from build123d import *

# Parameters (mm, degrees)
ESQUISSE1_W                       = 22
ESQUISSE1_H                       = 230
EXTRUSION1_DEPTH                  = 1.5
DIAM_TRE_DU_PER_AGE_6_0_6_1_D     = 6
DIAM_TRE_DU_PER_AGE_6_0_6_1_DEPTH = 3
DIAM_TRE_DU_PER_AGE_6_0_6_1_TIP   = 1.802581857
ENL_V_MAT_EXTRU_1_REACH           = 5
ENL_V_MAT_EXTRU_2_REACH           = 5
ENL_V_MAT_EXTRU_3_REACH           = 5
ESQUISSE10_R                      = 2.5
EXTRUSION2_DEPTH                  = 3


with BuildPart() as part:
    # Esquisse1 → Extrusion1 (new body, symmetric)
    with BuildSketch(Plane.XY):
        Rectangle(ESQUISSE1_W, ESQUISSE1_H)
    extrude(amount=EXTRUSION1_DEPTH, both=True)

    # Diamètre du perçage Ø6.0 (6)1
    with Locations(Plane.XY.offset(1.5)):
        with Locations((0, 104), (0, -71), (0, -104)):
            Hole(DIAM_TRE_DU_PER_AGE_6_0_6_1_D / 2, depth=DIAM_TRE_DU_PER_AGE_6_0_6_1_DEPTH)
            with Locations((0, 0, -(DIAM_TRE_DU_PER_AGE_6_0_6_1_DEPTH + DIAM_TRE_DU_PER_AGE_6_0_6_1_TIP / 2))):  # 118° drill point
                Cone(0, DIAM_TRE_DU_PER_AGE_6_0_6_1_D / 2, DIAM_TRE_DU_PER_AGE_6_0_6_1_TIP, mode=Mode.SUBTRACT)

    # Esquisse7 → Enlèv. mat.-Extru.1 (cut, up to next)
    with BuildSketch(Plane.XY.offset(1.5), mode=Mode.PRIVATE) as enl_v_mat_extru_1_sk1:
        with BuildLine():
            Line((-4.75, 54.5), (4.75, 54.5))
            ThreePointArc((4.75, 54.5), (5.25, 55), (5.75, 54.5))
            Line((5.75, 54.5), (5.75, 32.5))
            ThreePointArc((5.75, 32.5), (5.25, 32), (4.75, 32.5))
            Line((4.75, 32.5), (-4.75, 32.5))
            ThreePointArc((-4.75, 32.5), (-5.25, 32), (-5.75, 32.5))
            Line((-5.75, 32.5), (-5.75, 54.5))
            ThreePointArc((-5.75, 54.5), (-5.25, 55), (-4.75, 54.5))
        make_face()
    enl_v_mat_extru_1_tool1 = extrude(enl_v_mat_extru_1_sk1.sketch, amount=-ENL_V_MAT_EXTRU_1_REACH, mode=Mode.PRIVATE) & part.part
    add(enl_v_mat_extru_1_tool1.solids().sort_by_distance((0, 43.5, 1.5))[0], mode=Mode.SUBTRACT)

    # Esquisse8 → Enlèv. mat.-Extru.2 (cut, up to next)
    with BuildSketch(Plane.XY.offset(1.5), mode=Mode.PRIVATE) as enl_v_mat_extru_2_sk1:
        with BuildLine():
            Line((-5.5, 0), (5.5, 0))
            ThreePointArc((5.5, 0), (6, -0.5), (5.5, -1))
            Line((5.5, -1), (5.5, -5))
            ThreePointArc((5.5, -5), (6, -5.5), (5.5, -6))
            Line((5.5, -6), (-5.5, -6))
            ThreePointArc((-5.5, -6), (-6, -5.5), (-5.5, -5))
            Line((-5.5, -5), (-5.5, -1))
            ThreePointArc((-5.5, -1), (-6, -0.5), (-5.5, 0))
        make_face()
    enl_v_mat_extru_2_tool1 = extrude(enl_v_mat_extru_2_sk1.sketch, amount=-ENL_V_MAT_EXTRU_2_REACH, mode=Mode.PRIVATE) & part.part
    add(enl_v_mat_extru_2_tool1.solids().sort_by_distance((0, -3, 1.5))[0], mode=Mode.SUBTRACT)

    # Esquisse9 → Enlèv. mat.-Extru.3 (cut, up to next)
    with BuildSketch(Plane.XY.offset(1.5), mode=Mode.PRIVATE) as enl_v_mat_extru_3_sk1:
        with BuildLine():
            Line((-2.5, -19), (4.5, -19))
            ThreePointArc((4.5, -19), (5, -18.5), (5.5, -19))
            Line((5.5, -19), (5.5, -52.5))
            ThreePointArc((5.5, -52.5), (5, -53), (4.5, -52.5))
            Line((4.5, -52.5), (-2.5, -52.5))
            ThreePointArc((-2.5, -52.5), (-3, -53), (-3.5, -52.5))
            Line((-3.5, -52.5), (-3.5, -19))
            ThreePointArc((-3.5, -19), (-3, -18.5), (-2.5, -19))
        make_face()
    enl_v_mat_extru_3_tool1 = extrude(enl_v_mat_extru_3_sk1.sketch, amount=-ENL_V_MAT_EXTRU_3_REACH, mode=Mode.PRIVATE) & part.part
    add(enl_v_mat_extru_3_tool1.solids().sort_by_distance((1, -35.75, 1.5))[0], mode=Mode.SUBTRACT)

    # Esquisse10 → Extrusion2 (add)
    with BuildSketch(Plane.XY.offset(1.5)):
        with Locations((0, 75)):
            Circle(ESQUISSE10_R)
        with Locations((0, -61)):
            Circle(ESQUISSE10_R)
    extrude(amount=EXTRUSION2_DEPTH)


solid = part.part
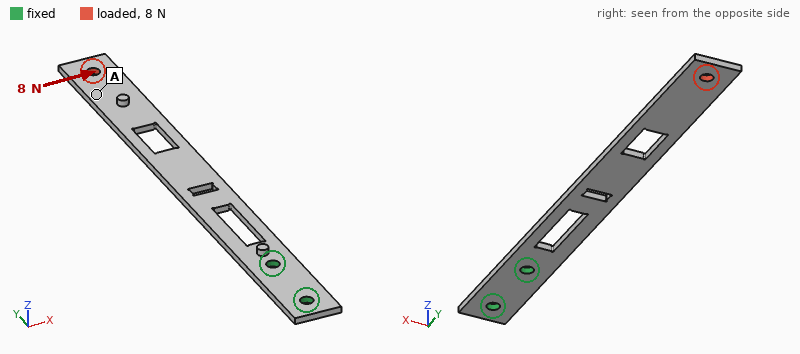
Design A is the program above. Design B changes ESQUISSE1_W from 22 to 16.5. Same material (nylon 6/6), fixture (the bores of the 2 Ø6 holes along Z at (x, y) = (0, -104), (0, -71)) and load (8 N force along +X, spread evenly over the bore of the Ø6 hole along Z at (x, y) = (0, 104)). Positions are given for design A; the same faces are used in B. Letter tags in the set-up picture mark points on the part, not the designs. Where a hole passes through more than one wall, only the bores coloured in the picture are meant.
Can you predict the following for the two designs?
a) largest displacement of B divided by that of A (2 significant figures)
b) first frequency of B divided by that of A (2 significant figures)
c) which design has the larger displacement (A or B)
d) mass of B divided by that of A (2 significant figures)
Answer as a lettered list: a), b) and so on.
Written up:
a) 2.6
b) 0.91
c) B
d) 0.71
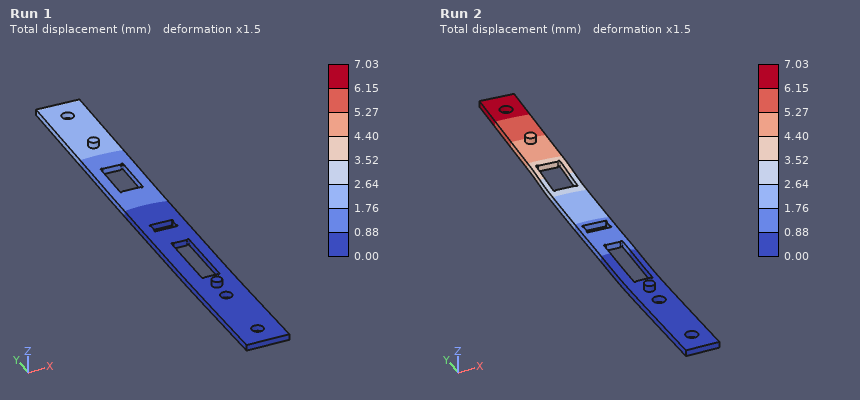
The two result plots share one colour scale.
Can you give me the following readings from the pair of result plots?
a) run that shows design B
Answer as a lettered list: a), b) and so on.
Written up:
a) Run 2
